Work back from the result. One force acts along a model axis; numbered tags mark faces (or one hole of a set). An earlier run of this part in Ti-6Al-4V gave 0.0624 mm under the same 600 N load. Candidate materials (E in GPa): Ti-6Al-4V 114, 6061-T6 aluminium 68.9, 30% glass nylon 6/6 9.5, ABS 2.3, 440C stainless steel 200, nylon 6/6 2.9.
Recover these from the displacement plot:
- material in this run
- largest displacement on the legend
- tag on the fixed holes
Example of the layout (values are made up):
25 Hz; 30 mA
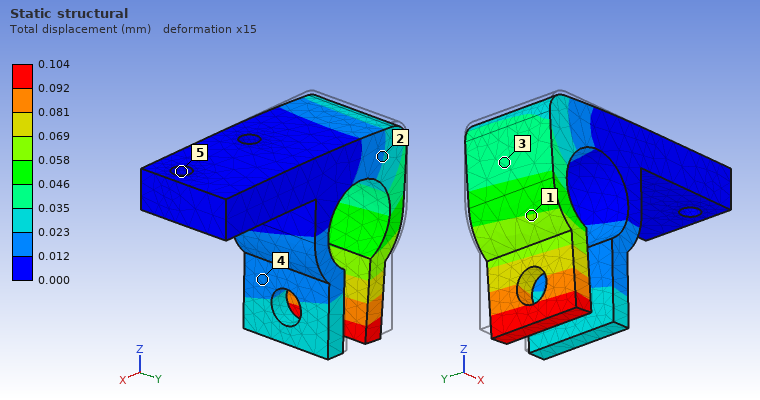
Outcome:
6061-T6 aluminium; 0.104 mm; 5
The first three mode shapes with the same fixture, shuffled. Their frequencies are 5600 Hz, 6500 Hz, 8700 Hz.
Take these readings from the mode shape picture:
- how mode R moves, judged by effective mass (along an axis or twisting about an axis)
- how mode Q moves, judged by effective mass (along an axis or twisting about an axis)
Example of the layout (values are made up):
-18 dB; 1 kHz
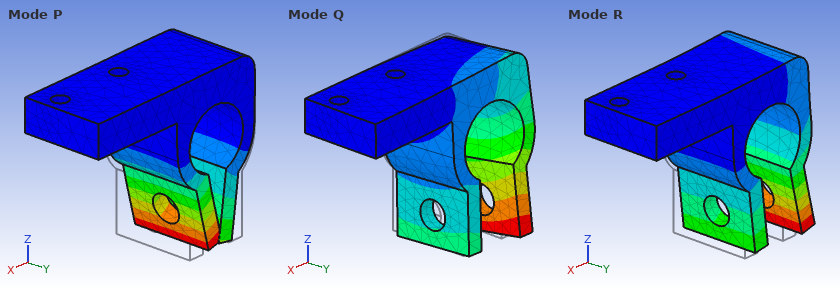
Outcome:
along X; along Y
